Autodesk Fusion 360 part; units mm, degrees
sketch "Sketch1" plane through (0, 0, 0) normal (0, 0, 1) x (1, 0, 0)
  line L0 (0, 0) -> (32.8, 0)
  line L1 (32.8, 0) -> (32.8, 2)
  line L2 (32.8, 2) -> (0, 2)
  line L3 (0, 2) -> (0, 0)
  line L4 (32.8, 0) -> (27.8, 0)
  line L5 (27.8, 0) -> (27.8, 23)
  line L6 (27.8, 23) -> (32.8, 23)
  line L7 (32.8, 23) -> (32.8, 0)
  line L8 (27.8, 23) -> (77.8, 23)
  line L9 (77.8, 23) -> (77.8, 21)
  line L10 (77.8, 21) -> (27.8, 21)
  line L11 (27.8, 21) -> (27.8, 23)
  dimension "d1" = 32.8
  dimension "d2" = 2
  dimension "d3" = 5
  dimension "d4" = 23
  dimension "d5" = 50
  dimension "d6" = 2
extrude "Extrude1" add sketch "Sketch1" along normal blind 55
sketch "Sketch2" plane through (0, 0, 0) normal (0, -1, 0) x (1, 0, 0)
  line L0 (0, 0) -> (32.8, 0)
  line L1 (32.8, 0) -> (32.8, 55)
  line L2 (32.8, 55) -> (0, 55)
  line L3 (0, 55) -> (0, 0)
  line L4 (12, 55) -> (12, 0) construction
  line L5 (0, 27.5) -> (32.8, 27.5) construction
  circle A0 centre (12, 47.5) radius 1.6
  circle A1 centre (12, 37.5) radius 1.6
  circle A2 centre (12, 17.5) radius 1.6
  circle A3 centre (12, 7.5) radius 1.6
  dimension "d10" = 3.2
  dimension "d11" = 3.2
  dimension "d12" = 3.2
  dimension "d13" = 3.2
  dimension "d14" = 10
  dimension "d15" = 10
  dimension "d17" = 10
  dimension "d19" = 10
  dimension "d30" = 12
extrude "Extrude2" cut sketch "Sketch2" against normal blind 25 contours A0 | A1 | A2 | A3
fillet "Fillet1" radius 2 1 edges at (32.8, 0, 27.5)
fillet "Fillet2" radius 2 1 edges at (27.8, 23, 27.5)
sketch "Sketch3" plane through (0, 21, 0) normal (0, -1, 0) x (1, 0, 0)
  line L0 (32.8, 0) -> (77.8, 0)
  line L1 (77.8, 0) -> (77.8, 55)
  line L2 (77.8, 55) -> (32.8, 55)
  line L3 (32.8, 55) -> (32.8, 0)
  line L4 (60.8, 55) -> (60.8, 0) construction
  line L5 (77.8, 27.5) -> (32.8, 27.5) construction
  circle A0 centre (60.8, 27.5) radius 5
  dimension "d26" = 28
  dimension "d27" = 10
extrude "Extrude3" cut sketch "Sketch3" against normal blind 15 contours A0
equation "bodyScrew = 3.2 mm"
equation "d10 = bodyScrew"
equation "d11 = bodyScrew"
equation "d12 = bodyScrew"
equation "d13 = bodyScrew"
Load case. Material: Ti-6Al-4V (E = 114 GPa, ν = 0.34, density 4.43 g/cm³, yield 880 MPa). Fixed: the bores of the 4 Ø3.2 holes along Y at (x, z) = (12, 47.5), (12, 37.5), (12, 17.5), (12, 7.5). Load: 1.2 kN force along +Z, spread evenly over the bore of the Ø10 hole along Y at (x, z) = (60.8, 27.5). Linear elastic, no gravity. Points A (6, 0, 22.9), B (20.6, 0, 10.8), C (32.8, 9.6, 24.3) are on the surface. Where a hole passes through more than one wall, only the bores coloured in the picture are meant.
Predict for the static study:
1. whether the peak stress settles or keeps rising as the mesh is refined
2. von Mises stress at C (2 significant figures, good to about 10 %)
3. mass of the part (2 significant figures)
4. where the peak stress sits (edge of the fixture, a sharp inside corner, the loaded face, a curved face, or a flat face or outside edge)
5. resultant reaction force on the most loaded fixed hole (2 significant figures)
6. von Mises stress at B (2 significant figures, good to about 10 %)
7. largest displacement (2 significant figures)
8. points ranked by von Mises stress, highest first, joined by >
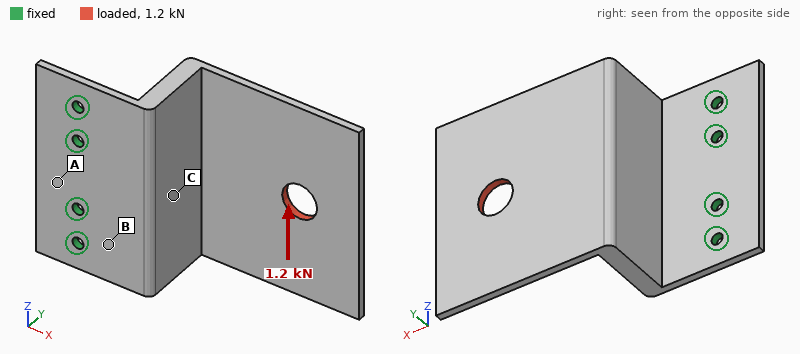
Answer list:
keeps rising
120 MPa
62 g
edge of the fixture
1.4 kN
66 MPa
0.47 mm
C > B > A
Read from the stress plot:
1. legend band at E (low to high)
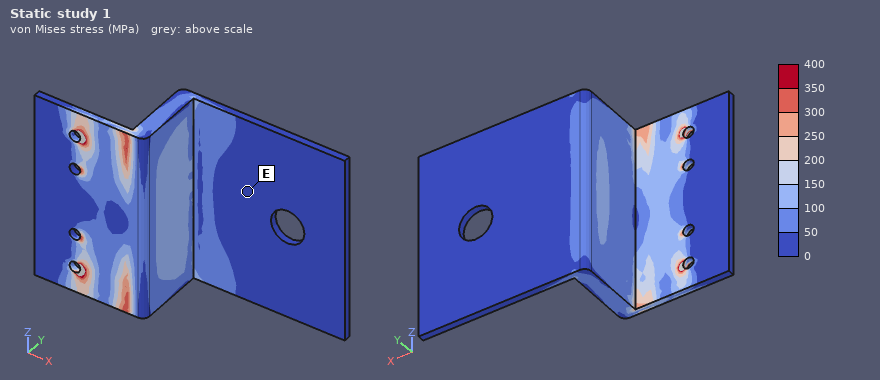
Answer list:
0 to 50 MPa
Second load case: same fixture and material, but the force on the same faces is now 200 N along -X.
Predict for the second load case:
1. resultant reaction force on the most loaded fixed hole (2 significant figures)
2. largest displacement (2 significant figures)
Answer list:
65 N
0.95 mm
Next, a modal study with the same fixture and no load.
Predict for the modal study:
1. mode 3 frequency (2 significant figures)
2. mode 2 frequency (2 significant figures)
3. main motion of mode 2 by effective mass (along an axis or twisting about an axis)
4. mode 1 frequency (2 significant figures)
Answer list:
1400 Hz
1300 Hz
along X
360 Hz
